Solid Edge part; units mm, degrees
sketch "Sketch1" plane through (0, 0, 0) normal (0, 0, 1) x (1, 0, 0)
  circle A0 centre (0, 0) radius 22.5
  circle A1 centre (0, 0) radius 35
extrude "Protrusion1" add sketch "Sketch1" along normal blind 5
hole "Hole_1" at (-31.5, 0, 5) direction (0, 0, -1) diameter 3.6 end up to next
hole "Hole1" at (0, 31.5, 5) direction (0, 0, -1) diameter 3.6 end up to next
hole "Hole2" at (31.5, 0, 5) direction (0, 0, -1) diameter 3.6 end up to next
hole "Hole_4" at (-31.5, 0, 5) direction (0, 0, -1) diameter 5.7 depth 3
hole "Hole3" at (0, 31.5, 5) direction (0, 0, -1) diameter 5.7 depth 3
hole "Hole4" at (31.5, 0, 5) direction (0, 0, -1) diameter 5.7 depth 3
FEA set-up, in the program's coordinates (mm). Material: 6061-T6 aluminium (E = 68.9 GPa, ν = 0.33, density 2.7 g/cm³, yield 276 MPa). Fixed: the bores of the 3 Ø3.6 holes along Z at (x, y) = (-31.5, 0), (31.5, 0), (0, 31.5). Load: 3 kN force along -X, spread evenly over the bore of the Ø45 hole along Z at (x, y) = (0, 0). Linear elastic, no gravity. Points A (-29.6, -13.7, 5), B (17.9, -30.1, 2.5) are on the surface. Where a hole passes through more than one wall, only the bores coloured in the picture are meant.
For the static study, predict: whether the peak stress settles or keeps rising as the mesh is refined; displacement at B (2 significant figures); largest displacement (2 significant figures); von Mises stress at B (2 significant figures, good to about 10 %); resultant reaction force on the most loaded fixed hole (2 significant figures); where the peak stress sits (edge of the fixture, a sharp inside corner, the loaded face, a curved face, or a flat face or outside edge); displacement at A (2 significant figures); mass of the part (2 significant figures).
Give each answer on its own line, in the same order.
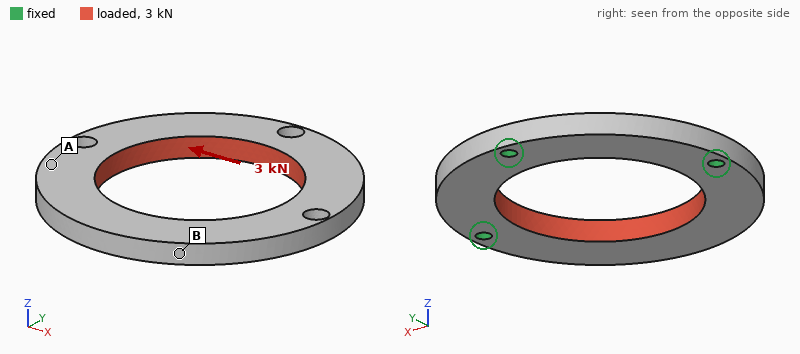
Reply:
keeps rising
27 µm
29 µm
19 MPa
1.2 kN
edge of the fixture
20 µm
30 g
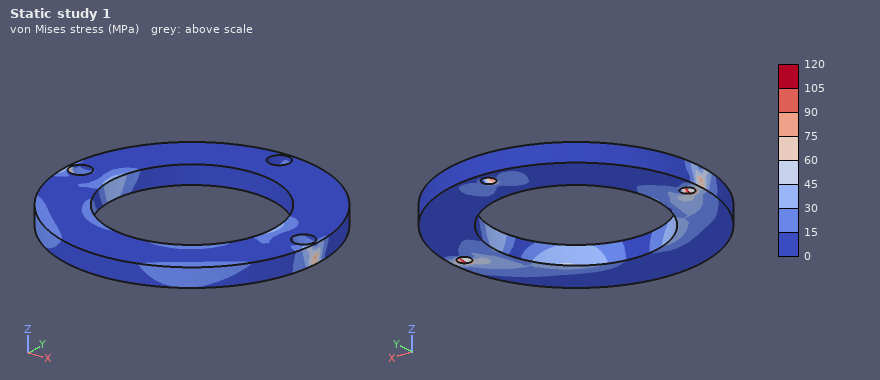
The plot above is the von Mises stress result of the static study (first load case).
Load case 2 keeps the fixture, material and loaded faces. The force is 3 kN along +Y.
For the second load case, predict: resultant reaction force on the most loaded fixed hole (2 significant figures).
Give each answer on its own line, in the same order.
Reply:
1.2 kN
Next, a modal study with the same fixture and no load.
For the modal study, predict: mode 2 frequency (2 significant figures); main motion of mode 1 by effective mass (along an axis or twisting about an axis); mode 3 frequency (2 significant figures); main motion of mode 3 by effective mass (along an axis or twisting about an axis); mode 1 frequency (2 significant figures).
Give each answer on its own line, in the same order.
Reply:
5400 Hz
along Z
7600 Hz
twisting about Y
1900 Hz
